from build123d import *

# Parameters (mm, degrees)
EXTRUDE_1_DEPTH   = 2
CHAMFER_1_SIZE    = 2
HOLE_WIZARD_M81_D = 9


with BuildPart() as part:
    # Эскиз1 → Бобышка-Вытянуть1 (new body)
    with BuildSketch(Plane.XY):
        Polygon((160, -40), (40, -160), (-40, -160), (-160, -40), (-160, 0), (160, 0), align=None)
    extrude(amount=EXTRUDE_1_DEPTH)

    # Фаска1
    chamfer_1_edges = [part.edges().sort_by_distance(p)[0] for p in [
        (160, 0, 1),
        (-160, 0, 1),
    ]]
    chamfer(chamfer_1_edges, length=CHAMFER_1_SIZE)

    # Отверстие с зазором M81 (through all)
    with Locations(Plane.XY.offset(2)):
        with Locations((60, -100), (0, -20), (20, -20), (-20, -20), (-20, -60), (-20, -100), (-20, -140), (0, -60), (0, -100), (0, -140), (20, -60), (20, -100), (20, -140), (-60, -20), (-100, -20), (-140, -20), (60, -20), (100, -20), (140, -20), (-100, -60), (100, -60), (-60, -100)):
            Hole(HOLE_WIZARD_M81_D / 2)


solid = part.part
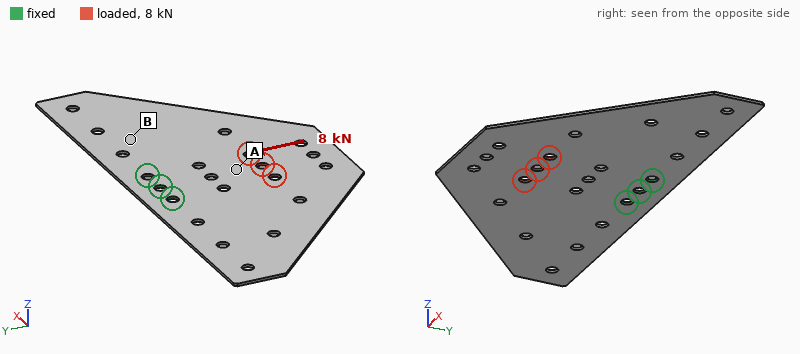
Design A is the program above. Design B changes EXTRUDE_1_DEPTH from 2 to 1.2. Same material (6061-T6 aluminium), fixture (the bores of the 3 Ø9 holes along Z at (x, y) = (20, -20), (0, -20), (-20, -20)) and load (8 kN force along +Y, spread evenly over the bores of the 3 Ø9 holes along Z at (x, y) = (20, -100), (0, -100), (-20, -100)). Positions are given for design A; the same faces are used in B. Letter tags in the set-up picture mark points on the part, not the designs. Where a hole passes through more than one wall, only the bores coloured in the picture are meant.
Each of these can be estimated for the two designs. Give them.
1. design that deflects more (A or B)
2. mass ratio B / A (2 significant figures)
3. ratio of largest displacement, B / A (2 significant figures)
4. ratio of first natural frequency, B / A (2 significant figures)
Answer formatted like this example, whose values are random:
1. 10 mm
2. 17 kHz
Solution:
1. B
2. 0.60
3. 1.7
4. 0.60
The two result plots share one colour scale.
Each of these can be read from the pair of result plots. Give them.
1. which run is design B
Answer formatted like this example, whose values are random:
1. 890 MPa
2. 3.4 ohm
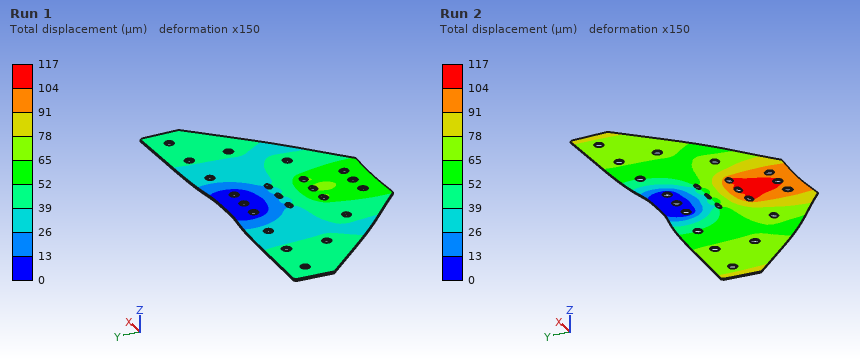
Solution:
1. Run 2
